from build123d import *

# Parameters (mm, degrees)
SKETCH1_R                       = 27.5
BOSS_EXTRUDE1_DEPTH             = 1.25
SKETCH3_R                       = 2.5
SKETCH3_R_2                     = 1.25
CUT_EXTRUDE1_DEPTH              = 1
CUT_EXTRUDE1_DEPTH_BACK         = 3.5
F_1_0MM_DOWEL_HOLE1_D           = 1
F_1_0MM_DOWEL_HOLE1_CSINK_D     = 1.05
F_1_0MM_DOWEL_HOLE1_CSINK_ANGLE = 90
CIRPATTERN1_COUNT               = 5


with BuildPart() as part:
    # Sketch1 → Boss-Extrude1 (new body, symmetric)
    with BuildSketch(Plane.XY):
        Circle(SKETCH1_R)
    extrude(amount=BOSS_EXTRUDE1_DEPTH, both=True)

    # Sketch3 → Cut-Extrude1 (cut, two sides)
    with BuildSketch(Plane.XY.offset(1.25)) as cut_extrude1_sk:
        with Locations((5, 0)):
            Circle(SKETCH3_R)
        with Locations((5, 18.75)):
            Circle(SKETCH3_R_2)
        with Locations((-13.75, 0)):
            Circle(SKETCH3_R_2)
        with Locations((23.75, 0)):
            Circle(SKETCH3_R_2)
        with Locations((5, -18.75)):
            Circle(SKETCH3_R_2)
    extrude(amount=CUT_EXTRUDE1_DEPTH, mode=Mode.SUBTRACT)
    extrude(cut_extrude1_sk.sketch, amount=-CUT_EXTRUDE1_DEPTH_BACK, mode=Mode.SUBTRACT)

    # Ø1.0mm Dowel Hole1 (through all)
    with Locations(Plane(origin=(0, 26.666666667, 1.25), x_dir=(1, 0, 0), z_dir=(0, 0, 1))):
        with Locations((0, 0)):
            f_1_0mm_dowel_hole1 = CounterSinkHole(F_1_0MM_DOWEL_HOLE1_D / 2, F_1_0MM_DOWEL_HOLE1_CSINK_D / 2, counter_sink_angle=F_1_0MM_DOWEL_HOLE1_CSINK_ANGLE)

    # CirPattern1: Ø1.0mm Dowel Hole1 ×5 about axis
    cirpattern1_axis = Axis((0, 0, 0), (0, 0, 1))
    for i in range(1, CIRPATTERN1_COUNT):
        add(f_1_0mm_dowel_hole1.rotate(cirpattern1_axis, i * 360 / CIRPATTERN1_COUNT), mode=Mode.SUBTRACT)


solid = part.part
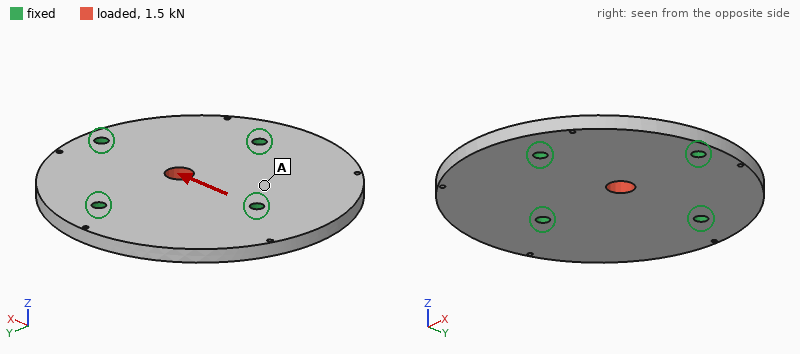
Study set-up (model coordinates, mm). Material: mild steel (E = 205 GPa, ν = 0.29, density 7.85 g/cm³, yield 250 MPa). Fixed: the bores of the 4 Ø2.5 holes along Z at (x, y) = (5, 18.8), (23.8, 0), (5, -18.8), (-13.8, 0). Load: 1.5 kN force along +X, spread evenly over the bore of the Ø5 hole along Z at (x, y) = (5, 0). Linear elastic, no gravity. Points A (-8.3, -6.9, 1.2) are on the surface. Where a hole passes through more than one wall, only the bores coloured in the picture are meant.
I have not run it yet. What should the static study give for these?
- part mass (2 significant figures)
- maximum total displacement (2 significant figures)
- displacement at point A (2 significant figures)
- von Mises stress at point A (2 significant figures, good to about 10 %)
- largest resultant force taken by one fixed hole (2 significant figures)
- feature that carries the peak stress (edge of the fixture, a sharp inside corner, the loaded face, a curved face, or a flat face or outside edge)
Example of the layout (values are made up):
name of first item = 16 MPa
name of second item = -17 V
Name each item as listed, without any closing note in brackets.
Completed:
part mass = 46 g
maximum total displacement = 2.0 µm
displacement at point A = 0.65 µm
von Mises stress at point A = 8.4 MPa
largest resultant force taken by one fixed hole = 500 N
feature that carries the peak stress = the loaded face
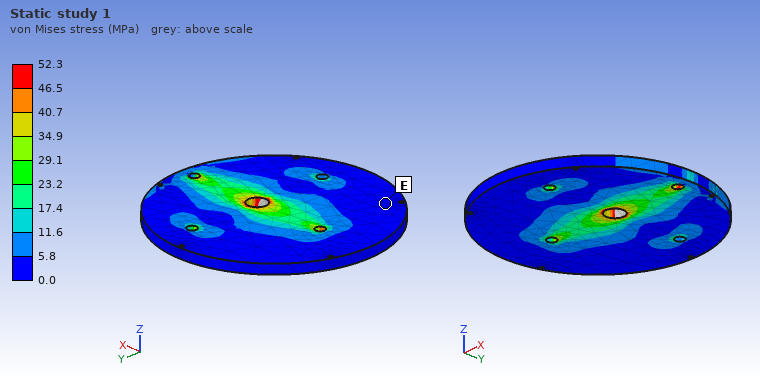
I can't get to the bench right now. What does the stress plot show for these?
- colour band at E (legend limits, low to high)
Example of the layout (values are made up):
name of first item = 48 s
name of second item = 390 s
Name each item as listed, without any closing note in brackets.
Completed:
colour band at E = 0.0 to 5.8 MPa
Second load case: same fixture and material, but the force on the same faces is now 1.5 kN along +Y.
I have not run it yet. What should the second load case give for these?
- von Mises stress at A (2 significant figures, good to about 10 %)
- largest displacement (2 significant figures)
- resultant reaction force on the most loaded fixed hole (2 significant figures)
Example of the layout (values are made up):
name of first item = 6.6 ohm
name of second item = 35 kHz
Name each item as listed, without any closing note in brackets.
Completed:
von Mises stress at A = 5.4 MPa
largest displacement = 2.0 µm
resultant reaction force on the most loaded fixed hole = 490 N
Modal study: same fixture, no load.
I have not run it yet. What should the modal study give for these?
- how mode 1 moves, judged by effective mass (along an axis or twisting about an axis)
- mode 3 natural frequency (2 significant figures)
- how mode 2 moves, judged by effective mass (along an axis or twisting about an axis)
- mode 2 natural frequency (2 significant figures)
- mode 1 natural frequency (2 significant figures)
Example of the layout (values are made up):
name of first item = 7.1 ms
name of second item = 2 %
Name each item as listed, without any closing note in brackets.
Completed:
how mode 1 moves, judged by effective mass = twisting about X
mode 3 natural frequency = 12 kHz
how mode 2 moves, judged by effective mass = along Z
mode 2 natural frequency = 7400 Hz
mode 1 natural frequency = 6600 Hz
